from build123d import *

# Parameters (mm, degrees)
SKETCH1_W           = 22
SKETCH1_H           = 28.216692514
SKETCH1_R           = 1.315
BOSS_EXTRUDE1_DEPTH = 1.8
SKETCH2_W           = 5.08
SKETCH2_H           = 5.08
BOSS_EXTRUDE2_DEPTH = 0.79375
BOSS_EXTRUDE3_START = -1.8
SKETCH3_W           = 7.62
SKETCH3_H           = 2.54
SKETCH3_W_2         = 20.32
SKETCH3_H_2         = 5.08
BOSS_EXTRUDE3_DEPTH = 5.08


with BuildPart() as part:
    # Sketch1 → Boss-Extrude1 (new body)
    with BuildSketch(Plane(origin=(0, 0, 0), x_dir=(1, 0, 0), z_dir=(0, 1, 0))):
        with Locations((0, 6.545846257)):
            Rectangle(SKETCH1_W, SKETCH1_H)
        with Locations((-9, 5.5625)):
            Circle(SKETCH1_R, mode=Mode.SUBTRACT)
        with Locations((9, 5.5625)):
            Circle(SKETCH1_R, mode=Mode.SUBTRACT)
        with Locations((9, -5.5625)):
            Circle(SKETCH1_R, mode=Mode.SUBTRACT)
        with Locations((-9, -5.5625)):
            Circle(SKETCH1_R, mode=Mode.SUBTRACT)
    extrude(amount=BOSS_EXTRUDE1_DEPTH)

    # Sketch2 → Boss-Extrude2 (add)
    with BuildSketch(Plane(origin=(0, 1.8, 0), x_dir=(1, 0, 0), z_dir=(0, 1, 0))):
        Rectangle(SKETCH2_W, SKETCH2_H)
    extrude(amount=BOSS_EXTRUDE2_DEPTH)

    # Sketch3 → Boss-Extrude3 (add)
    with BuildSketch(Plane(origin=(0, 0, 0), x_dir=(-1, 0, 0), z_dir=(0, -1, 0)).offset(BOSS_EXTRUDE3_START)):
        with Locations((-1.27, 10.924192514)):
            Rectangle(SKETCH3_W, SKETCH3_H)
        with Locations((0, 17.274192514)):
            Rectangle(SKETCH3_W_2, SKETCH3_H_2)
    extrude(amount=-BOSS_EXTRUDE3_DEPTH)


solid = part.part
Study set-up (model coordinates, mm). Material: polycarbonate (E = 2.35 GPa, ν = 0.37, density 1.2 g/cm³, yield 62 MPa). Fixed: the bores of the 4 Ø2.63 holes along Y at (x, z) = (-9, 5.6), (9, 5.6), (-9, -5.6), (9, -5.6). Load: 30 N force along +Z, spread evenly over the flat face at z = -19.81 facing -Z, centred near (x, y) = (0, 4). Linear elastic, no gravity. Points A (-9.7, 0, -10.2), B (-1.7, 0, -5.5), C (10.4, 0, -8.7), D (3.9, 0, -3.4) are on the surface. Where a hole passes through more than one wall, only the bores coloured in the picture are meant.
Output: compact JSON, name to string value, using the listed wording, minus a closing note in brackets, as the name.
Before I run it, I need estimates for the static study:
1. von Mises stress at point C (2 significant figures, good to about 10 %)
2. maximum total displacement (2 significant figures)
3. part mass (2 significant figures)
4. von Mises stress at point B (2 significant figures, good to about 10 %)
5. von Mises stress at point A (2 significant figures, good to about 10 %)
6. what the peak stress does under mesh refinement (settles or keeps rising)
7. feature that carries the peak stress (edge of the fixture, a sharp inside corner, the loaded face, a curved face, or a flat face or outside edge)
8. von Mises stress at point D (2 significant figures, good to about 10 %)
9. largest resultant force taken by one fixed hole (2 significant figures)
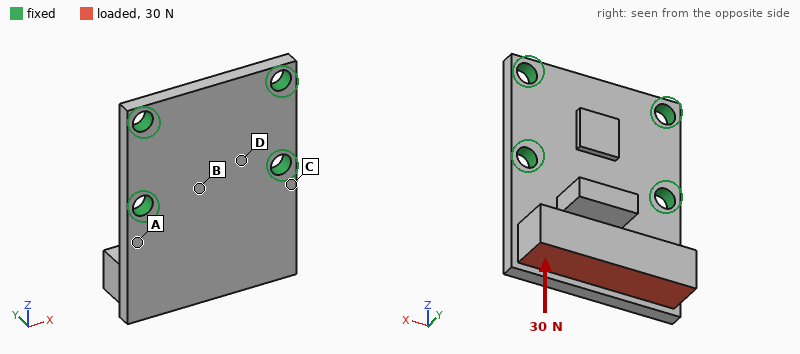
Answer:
{"von Mises stress at point C": "9.3 MPa", "maximum total displacement": "0.40 mm", "part mass": "2.1 g", "von Mises stress at point B": "3.7 MPa", "von Mises stress at point A": "8.2 MPa", "what the peak stress does under mesh refinement": "keeps rising", "feature that carries the peak stress": "edge of the fixture", "von Mises stress at point D": "1.9 MPa", "largest resultant force taken by one fixed hole": "12 N"}
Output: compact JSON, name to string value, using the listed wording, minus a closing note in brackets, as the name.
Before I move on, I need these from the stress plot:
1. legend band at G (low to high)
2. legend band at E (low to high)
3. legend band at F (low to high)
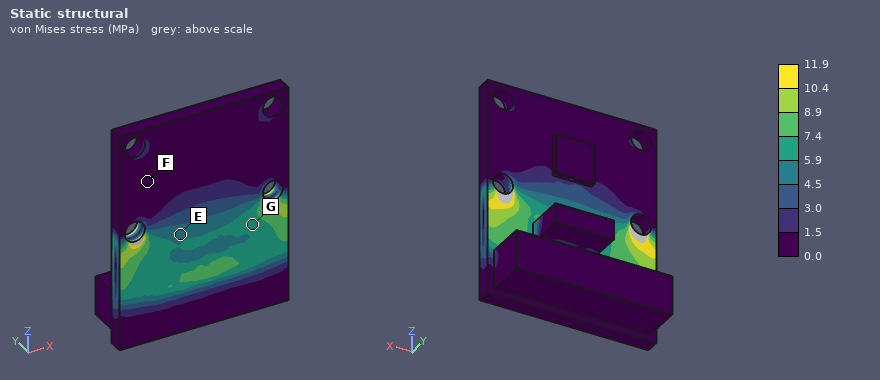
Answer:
{"legend band at G": "5.9 to 7.4 MPa", "legend band at E": "4.5 to 5.9 MPa", "legend band at F": "0.0 to 1.5 MPa"}
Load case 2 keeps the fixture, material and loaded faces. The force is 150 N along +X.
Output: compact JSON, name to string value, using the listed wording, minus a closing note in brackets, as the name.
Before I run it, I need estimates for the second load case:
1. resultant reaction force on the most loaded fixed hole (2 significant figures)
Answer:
{"resultant reaction force on the most loaded fixed hole": "140 N"}
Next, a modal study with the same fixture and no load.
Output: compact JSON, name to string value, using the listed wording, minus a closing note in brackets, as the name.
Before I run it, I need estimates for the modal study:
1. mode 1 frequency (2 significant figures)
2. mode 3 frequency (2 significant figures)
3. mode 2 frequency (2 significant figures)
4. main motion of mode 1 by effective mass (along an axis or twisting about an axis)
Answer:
{"mode 1 frequency": "1000 Hz", "mode 3 frequency": "5300 Hz", "mode 2 frequency": "3000 Hz", "main motion of mode 1 by effective mass": "along Y"}
